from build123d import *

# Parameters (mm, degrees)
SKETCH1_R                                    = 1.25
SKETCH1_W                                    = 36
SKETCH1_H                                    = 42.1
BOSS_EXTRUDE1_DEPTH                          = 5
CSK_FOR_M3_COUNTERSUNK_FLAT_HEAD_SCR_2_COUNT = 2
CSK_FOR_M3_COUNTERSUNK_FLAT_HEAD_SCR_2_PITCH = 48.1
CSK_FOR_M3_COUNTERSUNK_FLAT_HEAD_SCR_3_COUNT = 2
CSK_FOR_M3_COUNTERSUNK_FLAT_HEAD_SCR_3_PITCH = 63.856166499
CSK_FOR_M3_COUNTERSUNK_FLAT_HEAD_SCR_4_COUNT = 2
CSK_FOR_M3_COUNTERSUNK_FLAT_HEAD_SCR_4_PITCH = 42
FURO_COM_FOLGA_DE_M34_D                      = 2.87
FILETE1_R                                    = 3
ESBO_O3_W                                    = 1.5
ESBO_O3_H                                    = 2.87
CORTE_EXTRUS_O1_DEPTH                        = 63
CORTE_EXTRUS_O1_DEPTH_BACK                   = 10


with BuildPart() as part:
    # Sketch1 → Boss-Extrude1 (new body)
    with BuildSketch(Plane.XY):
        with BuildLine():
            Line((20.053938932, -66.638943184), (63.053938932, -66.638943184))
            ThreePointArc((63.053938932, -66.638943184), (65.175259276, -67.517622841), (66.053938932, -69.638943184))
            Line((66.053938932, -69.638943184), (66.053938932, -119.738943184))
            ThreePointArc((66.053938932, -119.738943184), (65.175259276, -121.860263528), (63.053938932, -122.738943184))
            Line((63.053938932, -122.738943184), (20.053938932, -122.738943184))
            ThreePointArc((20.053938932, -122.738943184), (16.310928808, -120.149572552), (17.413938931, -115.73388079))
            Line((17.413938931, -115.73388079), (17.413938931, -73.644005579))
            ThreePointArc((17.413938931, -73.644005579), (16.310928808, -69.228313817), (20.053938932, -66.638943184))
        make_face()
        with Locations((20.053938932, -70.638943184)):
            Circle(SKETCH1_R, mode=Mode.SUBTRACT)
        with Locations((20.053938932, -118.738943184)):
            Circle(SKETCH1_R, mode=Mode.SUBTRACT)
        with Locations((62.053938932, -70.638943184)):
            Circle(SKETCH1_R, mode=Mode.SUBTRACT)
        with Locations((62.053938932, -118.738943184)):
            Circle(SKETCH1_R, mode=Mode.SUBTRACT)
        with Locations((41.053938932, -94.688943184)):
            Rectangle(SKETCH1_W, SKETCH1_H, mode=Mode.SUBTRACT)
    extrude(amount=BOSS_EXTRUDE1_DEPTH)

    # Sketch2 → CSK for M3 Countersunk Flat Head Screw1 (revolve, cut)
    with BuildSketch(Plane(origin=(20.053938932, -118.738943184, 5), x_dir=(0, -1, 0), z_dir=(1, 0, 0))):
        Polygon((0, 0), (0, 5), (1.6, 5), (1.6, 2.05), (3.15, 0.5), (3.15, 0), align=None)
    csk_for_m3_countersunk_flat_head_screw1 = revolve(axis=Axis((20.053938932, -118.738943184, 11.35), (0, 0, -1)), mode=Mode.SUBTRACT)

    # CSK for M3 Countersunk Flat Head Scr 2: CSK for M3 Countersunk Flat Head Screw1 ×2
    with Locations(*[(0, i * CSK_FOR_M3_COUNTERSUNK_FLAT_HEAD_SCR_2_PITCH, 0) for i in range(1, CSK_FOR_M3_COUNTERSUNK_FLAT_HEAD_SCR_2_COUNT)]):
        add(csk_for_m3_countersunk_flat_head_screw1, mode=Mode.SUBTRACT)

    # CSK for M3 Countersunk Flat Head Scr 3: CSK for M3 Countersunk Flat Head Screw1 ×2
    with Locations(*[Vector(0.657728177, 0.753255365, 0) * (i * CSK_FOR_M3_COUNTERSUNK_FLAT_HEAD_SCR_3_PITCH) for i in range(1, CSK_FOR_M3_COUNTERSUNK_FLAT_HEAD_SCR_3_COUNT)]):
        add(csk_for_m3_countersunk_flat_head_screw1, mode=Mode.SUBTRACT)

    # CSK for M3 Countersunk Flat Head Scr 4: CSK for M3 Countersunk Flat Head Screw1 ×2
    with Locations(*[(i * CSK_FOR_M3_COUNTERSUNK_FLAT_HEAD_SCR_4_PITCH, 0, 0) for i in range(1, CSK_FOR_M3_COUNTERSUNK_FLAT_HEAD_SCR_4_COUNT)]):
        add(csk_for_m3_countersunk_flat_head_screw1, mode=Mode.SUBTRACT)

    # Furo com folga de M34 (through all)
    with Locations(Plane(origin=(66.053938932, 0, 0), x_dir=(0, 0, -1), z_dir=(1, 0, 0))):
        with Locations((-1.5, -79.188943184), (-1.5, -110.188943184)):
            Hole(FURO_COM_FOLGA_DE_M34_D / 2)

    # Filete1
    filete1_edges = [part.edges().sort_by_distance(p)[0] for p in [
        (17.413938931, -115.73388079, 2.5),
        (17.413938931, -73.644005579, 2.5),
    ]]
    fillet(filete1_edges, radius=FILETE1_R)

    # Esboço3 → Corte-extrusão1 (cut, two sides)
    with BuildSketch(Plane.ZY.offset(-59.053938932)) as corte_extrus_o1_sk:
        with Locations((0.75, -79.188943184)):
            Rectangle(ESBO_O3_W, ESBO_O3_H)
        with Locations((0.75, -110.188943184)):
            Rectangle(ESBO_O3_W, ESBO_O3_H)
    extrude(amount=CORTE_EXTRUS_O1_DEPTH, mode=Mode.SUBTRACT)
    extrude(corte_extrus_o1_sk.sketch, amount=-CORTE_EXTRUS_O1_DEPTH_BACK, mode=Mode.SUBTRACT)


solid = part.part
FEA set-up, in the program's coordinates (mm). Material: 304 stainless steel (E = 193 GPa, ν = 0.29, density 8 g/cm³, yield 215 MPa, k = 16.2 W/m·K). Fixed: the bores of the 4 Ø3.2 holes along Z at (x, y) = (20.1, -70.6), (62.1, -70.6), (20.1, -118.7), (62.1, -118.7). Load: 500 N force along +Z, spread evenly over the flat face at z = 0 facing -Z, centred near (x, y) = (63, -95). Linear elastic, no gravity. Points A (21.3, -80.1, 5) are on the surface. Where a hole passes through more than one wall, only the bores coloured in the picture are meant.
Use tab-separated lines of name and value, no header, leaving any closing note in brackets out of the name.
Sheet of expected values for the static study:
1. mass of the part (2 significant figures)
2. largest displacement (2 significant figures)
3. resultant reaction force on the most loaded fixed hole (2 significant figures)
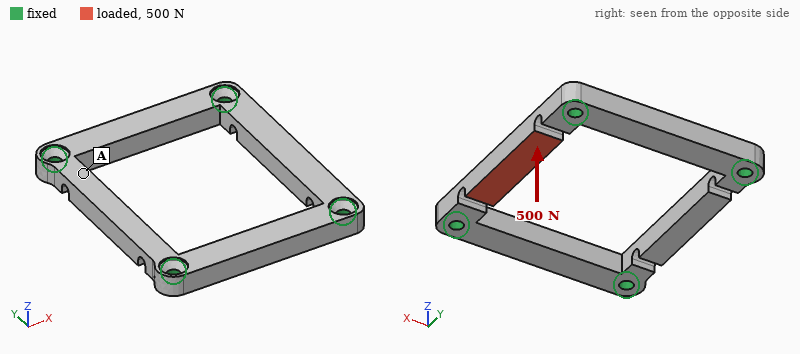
mass of the part	45 g
largest displacement	23 µm
resultant reaction force on the most loaded fixed hole	250 N
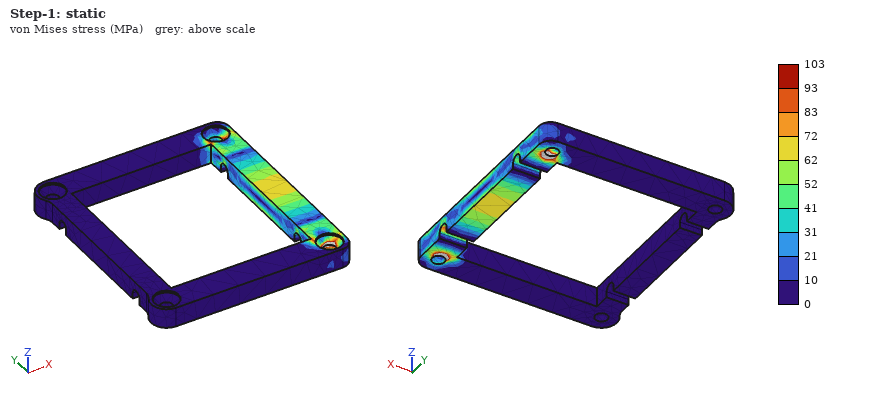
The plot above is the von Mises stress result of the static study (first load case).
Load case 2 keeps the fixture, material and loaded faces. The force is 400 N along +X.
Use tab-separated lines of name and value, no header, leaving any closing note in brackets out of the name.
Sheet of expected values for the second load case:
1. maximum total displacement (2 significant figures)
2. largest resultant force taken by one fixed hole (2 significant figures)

maximum total displacement	18 µm
largest resultant force taken by one fixed hole	200 N
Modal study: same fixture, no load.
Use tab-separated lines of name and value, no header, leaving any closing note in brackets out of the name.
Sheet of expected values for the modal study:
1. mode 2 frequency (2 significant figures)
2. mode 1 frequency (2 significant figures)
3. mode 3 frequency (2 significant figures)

mode 2 frequency	9200 Hz
mode 1 frequency	9000 Hz
mode 3 frequency	10 kHz
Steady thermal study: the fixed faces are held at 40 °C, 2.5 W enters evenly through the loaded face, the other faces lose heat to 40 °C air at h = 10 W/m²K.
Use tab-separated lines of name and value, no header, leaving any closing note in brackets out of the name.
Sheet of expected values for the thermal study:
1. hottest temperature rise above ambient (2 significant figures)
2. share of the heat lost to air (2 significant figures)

hottest temperature rise above ambient	47 K
share of the heat lost to air	11 %
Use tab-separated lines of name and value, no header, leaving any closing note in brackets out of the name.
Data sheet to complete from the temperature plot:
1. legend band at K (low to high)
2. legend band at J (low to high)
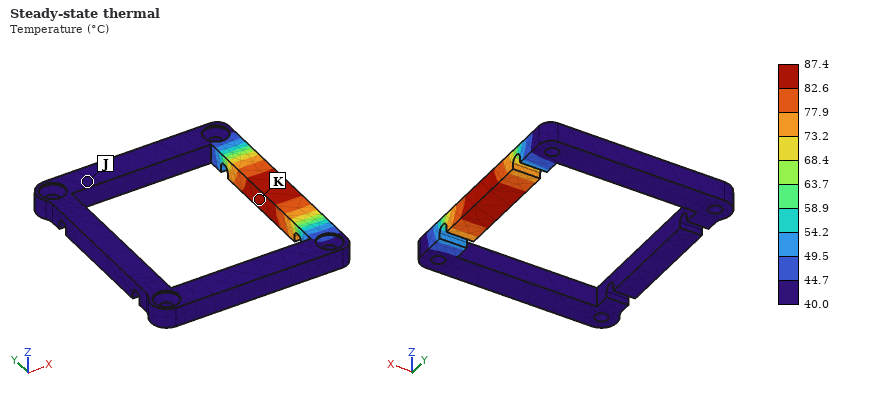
legend band at K	82.6 to 87.4 °C
legend band at J	40.0 to 44.7 °C
